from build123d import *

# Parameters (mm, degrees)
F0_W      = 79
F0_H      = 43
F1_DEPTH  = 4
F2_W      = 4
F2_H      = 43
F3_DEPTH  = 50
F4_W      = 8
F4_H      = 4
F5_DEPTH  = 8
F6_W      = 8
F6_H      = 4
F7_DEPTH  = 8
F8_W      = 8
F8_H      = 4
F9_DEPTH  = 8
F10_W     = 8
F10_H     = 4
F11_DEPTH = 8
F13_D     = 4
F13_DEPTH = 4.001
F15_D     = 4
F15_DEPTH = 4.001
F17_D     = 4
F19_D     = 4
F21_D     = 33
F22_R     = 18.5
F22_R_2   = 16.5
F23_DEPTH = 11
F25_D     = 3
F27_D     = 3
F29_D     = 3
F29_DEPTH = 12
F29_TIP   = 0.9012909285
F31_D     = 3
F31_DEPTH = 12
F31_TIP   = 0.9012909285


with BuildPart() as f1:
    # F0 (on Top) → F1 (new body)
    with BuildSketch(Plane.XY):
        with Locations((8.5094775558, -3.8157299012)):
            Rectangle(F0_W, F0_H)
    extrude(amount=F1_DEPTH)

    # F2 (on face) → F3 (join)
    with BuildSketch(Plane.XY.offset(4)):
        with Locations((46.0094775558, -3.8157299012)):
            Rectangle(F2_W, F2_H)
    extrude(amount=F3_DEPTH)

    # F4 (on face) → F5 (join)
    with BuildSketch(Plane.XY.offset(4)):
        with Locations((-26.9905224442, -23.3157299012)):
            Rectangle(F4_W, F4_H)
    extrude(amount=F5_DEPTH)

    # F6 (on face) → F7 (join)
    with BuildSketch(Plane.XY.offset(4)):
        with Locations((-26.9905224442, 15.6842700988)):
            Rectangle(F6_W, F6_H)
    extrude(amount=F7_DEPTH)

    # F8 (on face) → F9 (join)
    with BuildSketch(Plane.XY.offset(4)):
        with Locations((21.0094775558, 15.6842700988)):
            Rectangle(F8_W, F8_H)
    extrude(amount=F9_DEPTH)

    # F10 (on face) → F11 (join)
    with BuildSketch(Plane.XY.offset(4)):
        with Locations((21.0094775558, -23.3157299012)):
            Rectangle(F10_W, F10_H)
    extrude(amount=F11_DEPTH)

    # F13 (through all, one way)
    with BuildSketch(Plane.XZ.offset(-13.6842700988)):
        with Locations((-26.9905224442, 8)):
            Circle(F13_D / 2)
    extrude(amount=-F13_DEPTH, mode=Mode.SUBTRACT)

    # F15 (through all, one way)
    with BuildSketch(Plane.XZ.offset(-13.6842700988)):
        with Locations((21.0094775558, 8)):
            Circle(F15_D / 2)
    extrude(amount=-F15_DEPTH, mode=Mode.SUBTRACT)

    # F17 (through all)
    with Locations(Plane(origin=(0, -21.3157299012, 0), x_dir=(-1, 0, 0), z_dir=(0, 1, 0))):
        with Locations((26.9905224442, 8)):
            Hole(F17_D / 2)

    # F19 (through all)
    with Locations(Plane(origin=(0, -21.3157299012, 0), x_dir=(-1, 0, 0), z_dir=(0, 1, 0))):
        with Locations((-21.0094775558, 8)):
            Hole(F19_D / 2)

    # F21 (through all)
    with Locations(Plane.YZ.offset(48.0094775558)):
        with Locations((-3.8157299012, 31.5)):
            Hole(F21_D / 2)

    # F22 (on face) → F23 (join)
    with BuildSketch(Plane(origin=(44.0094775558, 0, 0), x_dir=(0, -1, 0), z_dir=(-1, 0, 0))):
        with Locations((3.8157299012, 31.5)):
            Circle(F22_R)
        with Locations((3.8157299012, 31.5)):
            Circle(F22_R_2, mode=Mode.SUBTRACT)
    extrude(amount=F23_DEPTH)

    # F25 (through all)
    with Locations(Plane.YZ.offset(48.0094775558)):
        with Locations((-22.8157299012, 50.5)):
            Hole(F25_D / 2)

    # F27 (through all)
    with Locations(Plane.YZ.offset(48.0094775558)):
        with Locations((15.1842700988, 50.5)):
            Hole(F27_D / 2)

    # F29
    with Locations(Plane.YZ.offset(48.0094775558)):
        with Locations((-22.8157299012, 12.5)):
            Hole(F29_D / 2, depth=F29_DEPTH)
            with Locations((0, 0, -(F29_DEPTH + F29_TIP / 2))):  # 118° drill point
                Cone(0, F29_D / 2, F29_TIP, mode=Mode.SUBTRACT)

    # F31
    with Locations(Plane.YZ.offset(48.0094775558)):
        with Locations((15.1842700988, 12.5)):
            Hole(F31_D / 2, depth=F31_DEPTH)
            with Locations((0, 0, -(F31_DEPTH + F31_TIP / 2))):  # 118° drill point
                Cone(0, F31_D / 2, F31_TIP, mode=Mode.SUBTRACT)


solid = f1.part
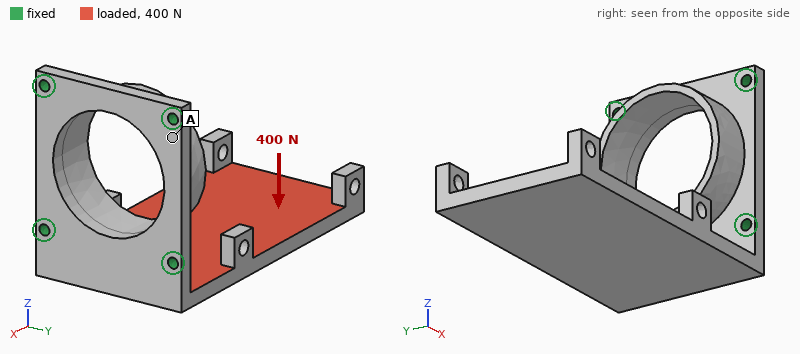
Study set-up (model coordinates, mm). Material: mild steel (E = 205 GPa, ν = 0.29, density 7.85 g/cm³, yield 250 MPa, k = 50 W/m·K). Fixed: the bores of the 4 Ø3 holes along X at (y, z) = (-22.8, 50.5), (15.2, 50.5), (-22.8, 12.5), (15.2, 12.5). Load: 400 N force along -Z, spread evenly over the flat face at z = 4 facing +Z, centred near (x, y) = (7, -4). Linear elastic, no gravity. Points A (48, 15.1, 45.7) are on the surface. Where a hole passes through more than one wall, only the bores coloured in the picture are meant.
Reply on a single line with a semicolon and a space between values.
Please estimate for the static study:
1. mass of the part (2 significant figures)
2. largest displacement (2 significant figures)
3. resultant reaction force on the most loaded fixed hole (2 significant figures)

170 g; 0.75 mm; 340 N
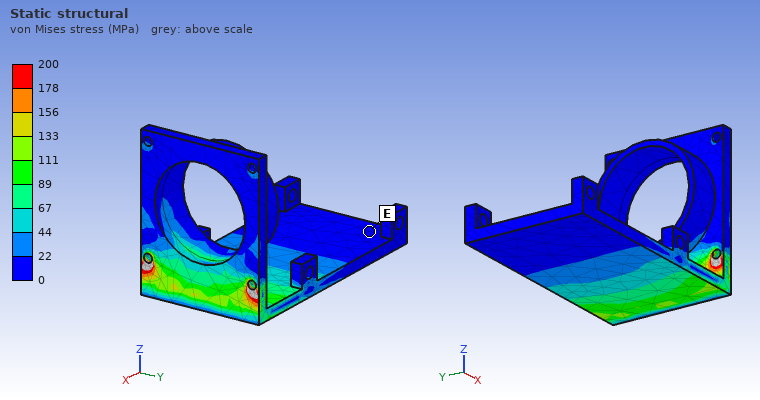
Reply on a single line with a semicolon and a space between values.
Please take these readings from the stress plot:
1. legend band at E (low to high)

0 to 22 MPa
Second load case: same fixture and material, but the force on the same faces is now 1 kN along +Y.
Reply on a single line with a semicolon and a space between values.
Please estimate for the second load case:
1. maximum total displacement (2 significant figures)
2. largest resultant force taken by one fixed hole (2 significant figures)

0.13 mm; 1.2 kN
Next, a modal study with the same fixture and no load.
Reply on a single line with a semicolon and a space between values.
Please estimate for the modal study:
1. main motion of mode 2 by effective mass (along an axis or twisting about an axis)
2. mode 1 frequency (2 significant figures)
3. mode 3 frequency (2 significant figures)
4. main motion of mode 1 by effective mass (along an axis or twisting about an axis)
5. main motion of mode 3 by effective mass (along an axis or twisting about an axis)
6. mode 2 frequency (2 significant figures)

along Y; 430 Hz; 2100 Hz; along Z; along Y; 1600 Hz
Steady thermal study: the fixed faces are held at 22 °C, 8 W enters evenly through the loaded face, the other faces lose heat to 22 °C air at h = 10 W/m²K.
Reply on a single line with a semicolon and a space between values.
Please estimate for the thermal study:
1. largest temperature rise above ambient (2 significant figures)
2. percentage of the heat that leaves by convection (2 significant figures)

39 K; 22 %
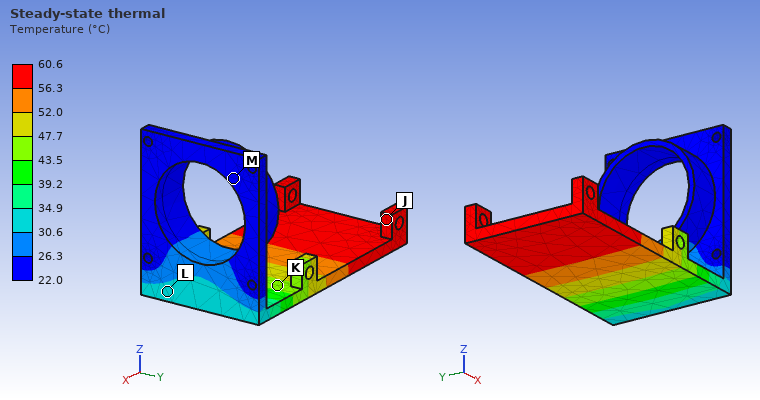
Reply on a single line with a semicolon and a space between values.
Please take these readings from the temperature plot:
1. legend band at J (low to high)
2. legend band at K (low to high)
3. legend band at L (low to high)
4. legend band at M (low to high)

56.3 to 60.6 °C; 43.5 to 47.7 °C; 30.6 to 34.9 °C; 22.0 to 26.3 °C
